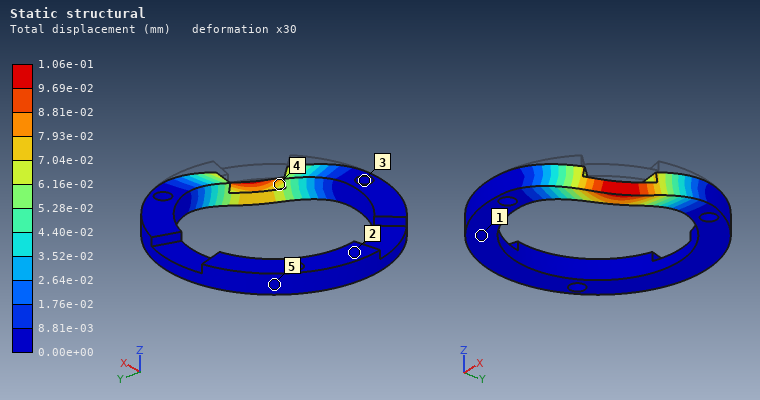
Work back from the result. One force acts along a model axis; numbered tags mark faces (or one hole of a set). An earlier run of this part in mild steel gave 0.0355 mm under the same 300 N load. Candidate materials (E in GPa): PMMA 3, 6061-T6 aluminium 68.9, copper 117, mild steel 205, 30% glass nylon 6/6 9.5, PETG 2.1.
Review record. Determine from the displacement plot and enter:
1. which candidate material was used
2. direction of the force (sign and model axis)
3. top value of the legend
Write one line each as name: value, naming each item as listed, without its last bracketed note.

which candidate material was used: 6061-T6 aluminium
direction of the force: -Z
top value of the legend: 1.06e-01 mm
